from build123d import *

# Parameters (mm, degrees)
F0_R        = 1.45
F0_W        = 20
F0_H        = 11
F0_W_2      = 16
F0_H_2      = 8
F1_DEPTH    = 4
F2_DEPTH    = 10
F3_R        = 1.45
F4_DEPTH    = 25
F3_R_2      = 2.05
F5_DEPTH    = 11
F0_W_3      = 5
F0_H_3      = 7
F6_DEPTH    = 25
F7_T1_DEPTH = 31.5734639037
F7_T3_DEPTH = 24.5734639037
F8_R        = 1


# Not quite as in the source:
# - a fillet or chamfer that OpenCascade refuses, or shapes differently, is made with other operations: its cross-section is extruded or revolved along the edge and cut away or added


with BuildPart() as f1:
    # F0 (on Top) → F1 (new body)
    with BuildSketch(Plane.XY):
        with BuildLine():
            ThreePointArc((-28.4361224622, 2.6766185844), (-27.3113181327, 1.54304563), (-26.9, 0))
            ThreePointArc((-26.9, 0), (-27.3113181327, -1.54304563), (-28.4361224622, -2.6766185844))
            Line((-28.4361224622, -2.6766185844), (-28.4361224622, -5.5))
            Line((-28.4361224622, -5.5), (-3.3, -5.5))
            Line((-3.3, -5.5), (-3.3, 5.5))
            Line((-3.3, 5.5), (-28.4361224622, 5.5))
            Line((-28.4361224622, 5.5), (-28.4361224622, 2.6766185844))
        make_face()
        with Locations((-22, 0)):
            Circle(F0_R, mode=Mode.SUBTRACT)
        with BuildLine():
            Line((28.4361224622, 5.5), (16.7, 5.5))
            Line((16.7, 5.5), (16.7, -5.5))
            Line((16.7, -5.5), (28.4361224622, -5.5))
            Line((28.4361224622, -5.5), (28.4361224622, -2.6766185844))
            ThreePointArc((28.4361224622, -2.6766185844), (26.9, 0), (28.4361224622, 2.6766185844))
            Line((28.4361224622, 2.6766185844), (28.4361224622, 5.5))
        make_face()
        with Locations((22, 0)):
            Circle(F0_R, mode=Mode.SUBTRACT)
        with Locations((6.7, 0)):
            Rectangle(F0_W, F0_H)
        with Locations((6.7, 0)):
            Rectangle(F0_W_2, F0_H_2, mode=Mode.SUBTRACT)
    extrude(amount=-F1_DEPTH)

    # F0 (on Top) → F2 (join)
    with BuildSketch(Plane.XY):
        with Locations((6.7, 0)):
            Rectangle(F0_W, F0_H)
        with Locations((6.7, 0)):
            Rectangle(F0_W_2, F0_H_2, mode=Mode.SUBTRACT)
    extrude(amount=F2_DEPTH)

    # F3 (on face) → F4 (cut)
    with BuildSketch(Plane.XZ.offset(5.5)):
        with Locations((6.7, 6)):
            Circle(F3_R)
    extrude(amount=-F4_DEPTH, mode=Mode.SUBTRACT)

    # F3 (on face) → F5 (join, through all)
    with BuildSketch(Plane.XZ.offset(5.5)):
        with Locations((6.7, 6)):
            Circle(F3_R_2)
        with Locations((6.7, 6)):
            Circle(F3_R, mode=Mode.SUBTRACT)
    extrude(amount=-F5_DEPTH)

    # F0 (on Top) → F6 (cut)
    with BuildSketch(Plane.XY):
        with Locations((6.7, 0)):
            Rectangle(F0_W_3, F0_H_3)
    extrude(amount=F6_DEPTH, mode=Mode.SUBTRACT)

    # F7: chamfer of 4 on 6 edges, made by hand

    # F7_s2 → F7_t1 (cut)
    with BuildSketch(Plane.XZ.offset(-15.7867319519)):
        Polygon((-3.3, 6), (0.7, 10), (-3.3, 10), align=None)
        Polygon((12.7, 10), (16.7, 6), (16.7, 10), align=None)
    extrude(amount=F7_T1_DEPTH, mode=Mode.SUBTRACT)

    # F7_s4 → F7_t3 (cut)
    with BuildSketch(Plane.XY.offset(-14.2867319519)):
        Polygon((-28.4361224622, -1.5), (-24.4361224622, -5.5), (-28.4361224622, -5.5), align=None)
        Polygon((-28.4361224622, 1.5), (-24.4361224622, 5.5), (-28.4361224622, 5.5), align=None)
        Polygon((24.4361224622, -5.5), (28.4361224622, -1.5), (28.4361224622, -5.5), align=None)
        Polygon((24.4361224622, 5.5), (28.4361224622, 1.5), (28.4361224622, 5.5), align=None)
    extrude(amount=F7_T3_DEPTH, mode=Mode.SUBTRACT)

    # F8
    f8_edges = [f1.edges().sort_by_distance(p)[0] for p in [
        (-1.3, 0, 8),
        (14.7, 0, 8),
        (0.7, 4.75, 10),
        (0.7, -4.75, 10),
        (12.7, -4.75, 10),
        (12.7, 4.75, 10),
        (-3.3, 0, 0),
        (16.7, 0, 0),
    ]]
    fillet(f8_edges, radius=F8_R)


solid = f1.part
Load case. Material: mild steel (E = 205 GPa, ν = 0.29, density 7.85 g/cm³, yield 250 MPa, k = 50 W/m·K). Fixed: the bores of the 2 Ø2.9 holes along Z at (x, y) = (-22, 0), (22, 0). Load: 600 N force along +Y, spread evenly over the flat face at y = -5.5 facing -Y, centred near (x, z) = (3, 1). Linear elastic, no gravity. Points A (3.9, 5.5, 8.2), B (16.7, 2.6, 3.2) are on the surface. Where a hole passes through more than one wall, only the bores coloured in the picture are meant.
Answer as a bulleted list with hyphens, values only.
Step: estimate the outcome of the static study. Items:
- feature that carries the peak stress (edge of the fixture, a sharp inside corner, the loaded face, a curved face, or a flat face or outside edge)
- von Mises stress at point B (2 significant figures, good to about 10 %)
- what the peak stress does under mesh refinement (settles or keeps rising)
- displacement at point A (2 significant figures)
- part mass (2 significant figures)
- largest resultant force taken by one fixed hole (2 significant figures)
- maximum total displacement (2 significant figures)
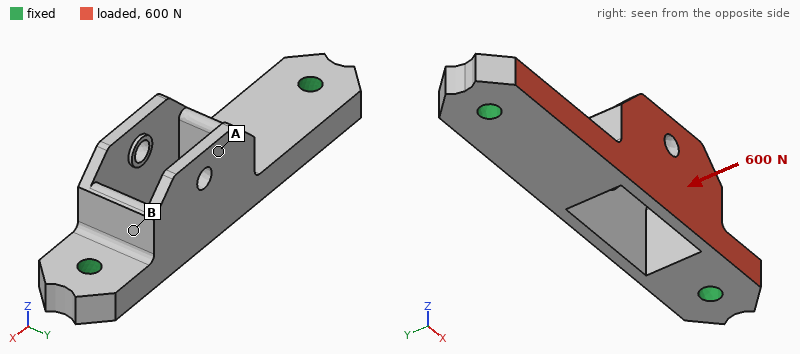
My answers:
- a sharp inside corner
- 32 MPa
- keeps rising
- 14 µm
- 20 g
- 310 N
- 32 µm
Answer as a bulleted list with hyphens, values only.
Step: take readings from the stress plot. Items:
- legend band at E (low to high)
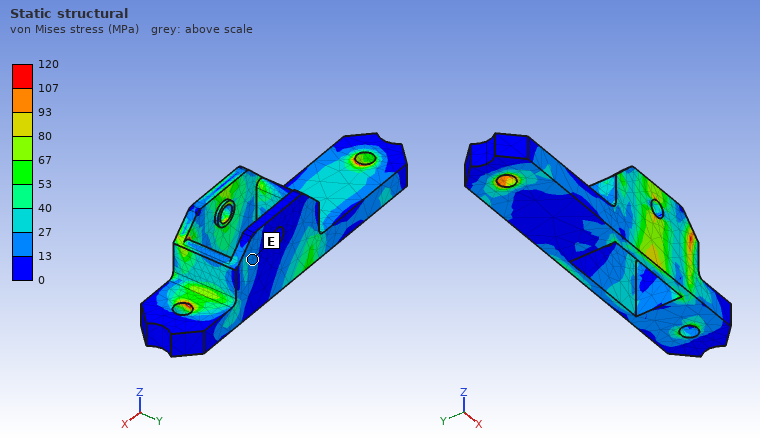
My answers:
- 13 to 27 MPa
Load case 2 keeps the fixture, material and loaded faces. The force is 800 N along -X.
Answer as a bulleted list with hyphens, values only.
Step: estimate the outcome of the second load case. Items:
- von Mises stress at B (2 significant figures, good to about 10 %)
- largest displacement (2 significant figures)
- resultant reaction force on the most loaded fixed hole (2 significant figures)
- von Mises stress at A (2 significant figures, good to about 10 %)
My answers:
- 15 MPa
- 8.0 µm
- 420 N
- 6.3 MPa
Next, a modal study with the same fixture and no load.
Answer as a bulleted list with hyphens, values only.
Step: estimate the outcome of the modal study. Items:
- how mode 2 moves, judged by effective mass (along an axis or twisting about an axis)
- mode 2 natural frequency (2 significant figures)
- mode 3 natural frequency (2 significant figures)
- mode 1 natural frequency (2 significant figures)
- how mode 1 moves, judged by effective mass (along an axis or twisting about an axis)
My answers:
- along Z
- 10 kHz
- 14 kHz
- 9200 Hz
- along Y
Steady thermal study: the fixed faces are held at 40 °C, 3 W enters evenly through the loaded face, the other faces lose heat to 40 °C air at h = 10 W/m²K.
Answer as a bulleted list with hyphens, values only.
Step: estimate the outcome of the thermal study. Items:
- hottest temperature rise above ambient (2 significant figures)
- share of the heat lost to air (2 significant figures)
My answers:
- 15 K
- 4.0 %
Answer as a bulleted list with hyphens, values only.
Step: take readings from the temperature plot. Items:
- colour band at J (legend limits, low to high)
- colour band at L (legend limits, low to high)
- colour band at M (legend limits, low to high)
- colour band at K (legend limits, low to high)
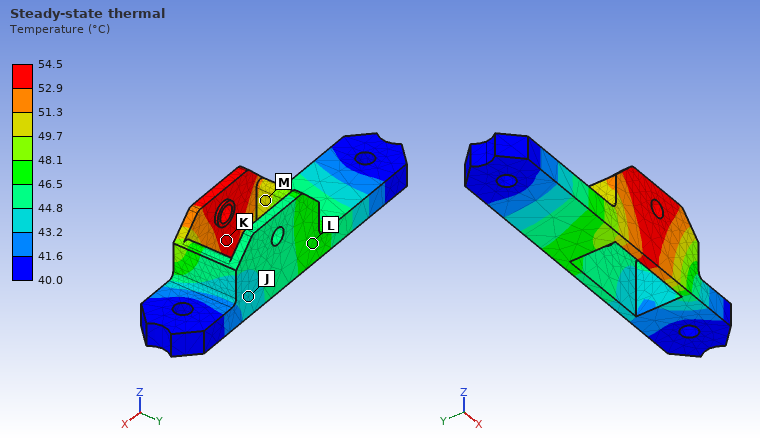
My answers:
- 43.2 to 44.8 °C
- 46.5 to 48.1 °C
- 49.7 to 51.3 °C
- 52.9 to 54.5 °C
